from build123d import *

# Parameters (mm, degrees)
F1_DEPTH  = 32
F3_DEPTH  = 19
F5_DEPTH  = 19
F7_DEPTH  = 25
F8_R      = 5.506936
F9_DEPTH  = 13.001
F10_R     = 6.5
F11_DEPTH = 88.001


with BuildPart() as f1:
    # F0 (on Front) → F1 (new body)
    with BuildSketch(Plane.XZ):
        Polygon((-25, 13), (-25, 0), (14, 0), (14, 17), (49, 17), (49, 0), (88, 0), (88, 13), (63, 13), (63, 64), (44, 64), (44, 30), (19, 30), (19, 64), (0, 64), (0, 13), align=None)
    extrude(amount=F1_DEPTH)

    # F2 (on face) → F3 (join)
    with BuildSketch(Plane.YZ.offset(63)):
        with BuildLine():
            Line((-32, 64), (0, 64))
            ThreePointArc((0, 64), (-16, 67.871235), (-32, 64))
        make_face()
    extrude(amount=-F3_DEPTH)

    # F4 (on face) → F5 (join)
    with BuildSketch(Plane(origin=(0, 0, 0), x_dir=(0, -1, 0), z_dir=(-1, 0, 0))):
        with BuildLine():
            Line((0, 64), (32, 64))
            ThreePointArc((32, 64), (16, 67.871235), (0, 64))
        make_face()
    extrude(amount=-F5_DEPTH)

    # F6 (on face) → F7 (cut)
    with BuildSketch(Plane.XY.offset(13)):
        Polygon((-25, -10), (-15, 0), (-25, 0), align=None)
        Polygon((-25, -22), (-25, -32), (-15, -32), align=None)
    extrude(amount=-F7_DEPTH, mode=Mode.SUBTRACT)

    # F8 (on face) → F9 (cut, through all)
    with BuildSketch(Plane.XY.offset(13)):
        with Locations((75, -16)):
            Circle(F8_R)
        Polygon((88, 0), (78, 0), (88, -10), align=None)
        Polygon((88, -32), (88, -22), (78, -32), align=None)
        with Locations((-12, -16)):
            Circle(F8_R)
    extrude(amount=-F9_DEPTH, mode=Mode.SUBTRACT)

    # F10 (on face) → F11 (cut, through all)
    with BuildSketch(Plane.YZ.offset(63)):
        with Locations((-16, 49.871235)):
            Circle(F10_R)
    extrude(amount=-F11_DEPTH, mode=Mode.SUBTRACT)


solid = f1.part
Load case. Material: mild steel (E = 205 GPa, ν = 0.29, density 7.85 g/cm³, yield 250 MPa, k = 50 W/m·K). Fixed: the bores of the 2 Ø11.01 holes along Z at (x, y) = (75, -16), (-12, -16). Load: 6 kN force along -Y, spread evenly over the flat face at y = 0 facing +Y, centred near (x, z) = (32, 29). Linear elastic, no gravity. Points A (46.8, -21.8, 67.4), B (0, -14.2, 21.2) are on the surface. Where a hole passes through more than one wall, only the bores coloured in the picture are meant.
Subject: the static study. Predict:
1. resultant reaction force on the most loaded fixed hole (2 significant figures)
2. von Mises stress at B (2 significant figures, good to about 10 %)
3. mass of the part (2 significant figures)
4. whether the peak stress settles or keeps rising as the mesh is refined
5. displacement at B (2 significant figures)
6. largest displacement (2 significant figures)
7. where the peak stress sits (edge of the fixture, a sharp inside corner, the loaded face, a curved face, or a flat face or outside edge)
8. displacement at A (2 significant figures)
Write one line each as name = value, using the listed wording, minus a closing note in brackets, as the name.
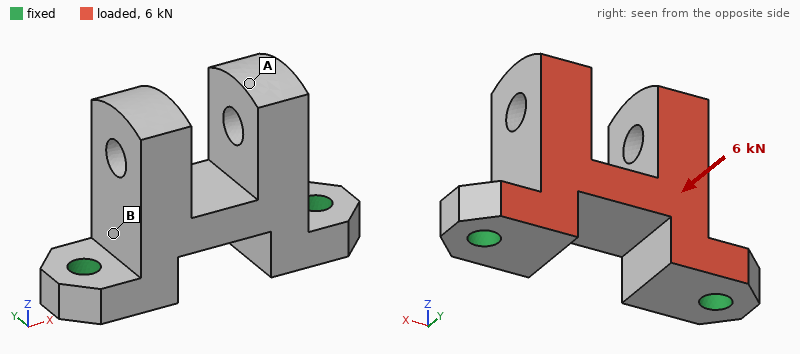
resultant reaction force on the most loaded fixed hole = 3.0 kN
von Mises stress at B = 19 MPa
mass of the part = 760 g
whether the peak stress settles or keeps rising as the mesh is refined = keeps rising
displacement at B = 11 µm
largest displacement = 44 µm
where the peak stress sits = edge of the fixture
displacement at A = 44 µm
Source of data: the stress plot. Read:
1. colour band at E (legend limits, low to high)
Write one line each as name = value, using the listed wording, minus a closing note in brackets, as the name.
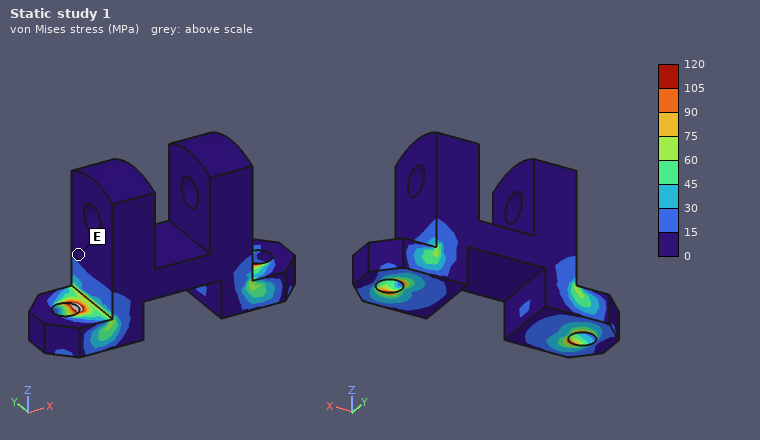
colour band at E = 0 to 15 MPa
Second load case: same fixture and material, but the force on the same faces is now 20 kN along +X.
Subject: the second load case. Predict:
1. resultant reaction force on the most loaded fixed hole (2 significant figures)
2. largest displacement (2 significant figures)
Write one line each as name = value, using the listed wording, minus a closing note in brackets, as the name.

resultant reaction force on the most loaded fixed hole = 12 kN
largest displacement = 53 µm
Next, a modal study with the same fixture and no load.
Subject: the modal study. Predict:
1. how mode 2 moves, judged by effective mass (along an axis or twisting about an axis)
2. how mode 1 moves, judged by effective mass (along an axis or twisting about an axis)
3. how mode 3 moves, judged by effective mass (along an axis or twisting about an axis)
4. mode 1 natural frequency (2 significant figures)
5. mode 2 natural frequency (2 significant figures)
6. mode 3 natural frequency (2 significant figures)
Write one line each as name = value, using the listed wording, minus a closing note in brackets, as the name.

how mode 2 moves, judged by effective mass = twisting about Z
how mode 1 moves, judged by effective mass = along Y
how mode 3 moves, judged by effective mass = along X
mode 1 natural frequency = 2600 Hz
mode 2 natural frequency = 4300 Hz
mode 3 natural frequency = 5100 Hz
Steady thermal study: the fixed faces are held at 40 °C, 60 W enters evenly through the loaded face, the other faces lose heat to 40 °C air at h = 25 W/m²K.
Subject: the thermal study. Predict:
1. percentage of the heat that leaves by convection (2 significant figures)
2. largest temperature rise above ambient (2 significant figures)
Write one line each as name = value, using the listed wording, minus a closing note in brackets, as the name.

percentage of the heat that leaves by convection = 17 %
largest temperature rise above ambient = 39 K
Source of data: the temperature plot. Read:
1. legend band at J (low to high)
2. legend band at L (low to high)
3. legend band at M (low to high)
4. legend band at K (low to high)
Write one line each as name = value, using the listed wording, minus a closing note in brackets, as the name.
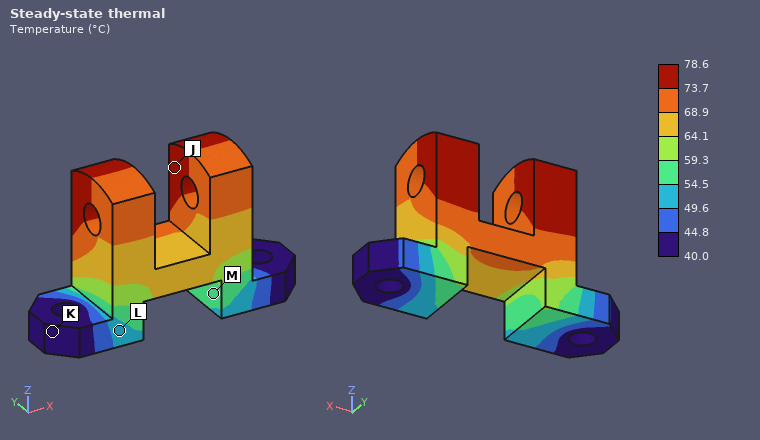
legend band at J = 73.7 to 78.6 °C
legend band at L = 49.6 to 54.5 °C
legend band at M = 54.5 to 59.3 °C
legend band at K = 40.0 to 44.8 °C
